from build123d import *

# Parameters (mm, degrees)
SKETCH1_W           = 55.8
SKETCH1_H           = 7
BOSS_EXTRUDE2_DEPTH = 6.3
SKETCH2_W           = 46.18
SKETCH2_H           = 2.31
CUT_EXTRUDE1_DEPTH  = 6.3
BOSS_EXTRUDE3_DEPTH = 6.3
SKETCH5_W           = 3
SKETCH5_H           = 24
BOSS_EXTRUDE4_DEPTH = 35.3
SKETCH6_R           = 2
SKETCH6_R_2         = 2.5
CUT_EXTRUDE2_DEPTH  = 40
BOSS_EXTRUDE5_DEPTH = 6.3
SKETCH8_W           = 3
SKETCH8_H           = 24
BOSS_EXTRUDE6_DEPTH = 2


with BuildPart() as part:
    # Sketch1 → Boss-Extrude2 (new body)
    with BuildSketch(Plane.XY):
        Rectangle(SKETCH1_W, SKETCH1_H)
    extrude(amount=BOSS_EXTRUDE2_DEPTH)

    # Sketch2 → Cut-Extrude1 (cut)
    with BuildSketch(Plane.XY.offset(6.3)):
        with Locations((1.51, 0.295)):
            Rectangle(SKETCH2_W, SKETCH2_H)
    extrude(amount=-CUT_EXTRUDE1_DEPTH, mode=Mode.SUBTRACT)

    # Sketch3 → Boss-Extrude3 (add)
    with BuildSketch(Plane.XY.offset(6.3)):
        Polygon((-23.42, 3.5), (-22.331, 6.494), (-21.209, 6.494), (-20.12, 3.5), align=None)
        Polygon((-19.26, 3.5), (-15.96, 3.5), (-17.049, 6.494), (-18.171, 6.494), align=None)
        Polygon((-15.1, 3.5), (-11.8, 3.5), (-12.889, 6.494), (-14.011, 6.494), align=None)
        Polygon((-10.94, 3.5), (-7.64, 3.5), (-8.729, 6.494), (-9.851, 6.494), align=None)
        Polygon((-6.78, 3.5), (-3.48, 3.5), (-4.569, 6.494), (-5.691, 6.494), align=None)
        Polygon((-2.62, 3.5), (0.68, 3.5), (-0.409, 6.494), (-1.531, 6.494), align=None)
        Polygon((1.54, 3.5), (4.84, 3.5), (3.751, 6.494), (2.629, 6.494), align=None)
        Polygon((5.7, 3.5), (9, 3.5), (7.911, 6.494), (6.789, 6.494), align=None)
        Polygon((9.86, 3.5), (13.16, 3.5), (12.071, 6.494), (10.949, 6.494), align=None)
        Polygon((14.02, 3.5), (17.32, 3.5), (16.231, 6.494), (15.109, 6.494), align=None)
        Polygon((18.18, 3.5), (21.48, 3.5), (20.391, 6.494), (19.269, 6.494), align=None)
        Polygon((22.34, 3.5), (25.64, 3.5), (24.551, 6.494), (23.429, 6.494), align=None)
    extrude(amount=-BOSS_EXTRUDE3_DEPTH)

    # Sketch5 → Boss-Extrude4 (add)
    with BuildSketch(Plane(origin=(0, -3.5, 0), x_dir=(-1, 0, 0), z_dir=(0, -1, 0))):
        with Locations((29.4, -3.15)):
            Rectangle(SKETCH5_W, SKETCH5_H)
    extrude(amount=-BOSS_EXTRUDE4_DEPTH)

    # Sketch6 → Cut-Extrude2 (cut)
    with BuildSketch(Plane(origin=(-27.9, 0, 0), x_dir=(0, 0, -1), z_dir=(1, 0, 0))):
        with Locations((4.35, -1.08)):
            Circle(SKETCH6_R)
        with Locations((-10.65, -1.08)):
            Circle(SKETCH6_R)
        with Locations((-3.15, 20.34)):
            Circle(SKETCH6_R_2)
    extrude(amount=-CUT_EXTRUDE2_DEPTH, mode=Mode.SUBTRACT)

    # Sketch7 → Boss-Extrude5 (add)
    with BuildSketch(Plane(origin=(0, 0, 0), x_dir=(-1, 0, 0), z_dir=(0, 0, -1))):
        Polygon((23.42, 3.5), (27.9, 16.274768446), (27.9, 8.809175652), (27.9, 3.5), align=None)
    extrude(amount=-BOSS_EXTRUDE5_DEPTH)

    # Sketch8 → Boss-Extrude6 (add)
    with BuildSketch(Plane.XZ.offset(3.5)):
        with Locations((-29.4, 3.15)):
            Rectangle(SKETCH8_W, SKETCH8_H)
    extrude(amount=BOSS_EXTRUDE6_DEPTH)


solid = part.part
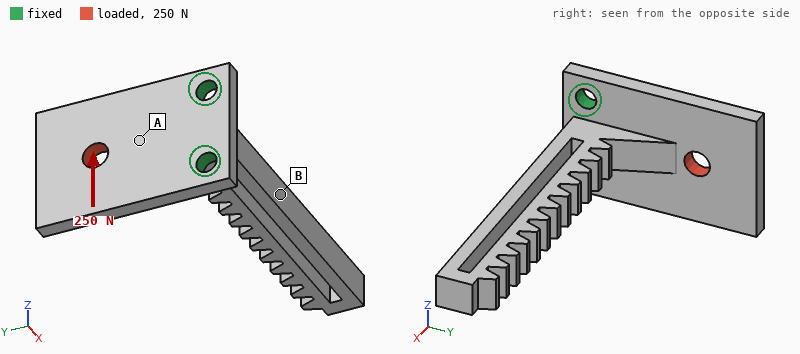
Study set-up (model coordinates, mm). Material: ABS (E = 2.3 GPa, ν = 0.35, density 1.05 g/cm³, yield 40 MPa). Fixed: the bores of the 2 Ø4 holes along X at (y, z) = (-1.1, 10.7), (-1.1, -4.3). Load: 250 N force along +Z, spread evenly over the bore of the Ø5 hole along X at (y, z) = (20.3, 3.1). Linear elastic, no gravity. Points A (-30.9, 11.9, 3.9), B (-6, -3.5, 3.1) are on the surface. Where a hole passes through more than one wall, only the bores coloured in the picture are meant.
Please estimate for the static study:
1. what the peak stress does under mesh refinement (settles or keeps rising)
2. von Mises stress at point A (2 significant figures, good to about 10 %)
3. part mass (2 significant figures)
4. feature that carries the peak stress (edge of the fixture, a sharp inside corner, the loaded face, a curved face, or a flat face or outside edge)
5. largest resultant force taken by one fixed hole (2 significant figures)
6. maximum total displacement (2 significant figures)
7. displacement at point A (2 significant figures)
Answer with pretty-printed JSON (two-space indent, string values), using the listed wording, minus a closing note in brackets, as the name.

{
  "what the peak stress does under mesh refinement": "keeps rising",
  "von Mises stress at point A": "9.8 MPa",
  "part mass": "5.3 g",
  "feature that carries the peak stress": "edge of the fixture",
  "largest resultant force taken by one fixed hole": "330 N",
  "maximum total displacement": "0.31 mm",
  "displacement at point A": "0.10 mm"
}
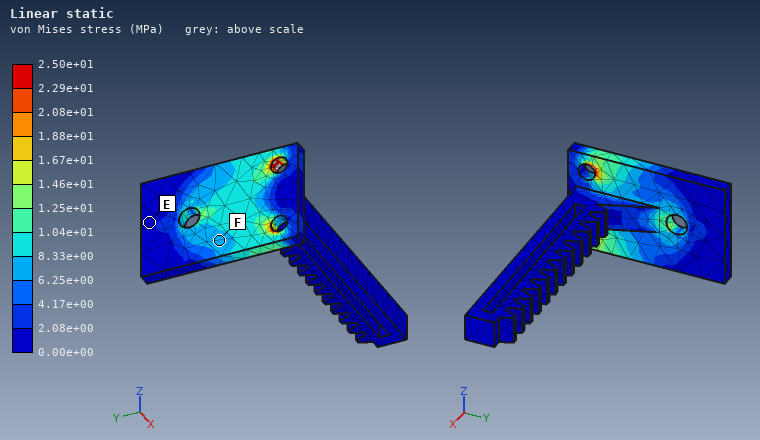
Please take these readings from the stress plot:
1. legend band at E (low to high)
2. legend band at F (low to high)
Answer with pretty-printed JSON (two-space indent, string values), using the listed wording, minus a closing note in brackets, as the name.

{
  "legend band at E": "0.00e+00 to 2.08e+00 MPa",
  "legend band at F": "6.25e+00 to 8.33e+00 MPa"
}
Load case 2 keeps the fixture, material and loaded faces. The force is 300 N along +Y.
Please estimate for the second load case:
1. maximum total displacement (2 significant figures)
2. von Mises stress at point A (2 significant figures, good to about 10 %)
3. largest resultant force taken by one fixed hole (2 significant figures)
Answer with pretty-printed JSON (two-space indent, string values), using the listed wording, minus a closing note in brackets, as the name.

{
  "maximum total displacement": "0.11 mm",
  "von Mises stress at point A": "6.0 MPa",
  "largest resultant force taken by one fixed hole": "150 N"
}
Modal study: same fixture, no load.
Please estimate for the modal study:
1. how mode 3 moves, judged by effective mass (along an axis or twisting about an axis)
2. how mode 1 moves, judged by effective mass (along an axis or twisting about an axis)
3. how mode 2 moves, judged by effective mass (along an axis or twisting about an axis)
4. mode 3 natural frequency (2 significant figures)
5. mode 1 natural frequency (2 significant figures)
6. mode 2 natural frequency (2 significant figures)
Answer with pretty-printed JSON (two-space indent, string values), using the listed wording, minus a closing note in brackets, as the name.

{
  "how mode 3 moves, judged by effective mass": "along X",
  "how mode 1 moves, judged by effective mass": "along Y",
  "how mode 2 moves, judged by effective mass": "along Z",
  "mode 3 natural frequency": "950 Hz",
  "mode 1 natural frequency": "290 Hz",
  "mode 2 natural frequency": "420 Hz"
}
